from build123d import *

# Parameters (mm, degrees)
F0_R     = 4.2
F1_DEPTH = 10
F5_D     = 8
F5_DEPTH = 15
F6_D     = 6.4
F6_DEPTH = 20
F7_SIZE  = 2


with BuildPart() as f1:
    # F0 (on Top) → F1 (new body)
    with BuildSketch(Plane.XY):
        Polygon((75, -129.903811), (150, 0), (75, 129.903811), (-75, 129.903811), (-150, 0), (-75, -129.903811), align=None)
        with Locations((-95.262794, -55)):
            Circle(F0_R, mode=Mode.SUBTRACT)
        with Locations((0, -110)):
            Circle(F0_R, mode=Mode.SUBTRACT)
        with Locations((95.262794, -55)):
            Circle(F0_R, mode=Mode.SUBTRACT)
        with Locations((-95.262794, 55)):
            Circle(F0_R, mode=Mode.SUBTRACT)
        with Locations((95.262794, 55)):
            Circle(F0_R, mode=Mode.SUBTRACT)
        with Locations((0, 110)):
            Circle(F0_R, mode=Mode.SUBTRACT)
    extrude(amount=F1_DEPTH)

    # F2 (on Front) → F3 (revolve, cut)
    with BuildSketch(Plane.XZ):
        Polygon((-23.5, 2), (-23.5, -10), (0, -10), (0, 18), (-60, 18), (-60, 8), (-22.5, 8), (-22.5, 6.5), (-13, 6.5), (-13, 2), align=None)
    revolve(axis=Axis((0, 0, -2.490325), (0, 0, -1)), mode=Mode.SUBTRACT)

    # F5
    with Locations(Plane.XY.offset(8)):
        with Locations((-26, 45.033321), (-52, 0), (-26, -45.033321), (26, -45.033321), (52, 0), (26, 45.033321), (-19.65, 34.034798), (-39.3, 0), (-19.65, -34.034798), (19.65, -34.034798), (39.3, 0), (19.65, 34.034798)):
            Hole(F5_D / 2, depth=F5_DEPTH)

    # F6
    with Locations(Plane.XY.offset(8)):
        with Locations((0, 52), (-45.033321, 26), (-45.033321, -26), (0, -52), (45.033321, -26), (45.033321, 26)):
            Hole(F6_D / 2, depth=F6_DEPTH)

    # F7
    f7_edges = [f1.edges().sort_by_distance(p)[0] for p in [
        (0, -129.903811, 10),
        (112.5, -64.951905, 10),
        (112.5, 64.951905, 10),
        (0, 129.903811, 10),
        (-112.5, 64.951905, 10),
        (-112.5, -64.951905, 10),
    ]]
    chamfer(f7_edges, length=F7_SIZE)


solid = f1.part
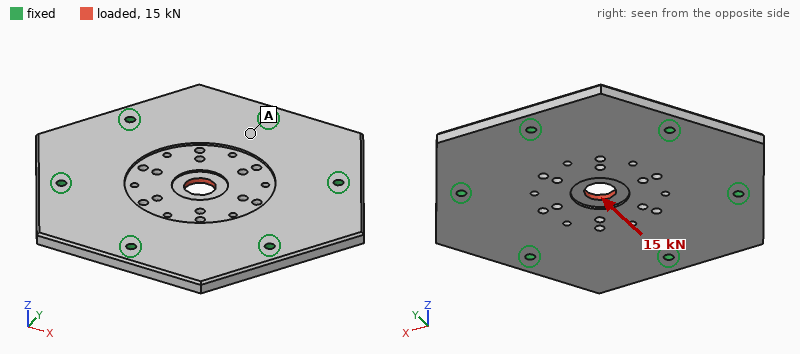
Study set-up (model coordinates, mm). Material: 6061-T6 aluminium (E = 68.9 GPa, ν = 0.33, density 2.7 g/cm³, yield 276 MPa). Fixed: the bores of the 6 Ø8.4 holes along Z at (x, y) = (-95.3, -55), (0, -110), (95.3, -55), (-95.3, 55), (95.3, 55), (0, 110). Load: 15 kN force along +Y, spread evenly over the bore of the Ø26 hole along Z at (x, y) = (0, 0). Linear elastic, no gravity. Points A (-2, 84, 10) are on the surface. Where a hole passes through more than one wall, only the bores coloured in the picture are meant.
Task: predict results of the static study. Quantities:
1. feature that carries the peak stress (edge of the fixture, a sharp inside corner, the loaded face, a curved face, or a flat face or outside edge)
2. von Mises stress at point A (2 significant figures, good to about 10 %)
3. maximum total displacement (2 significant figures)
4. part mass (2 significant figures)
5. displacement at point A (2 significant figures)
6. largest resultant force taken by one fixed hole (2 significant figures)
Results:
the loaded face
8.5 MPa
22 µm
1.5 kg
3.7 µm
3.7 kN
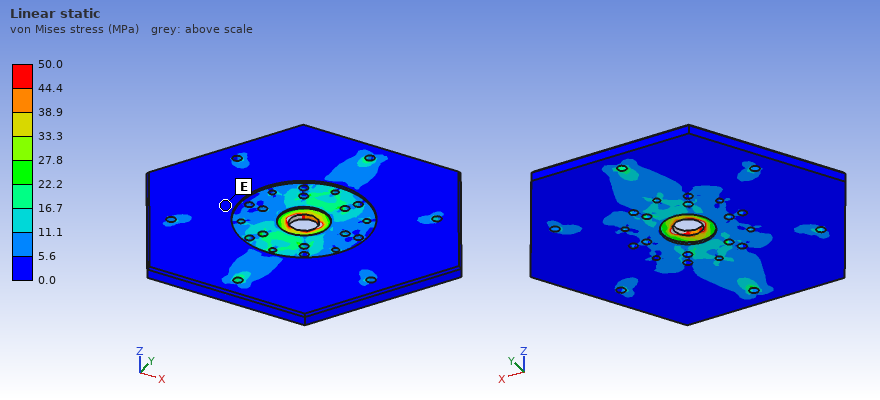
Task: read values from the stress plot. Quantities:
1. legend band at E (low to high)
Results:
0.0 to 5.6 MPa
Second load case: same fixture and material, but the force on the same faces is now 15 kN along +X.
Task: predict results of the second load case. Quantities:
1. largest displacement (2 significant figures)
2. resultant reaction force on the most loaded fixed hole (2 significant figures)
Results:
22 µm
3.3 kN
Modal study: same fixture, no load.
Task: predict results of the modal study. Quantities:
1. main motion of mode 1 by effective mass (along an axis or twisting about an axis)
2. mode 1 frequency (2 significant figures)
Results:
along Z
1600 Hz
